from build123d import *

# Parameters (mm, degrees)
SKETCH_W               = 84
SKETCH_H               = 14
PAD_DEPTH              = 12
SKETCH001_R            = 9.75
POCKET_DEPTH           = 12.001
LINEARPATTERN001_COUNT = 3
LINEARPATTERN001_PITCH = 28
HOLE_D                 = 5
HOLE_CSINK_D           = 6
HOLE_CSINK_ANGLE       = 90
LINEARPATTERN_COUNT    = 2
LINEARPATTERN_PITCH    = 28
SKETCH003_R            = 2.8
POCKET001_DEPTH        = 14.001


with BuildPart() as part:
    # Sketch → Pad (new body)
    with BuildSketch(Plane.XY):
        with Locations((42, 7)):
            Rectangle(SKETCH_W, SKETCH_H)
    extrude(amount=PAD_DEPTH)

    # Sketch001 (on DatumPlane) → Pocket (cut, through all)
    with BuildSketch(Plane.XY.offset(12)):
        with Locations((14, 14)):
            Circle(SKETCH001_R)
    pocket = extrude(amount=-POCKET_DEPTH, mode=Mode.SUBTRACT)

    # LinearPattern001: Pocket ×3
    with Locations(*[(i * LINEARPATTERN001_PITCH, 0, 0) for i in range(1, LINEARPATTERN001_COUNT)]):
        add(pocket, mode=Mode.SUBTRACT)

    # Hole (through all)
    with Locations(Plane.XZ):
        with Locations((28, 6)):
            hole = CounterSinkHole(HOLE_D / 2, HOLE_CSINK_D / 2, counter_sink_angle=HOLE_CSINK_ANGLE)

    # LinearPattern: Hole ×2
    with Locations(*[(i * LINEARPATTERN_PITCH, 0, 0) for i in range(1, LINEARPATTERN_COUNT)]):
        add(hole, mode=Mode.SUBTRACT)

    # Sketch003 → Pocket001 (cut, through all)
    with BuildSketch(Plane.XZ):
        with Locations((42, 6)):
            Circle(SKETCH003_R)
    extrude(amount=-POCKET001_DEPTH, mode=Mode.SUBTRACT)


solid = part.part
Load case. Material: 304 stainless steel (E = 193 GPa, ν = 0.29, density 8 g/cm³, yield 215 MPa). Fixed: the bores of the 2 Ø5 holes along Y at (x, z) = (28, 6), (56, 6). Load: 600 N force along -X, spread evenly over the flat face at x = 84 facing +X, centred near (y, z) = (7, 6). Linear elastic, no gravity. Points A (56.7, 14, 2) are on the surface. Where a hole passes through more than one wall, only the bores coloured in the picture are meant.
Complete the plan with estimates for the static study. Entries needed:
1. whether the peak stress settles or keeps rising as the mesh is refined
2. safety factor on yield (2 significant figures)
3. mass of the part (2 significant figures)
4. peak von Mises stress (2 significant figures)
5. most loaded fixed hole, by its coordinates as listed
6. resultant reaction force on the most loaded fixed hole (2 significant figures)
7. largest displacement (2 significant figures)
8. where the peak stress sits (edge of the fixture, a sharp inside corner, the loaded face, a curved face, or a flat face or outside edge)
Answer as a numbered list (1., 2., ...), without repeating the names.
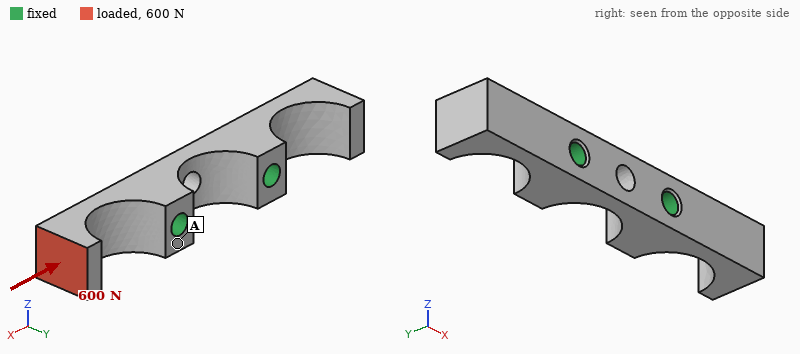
1. settles
2. 2.2
3. 65 g
4. 98 MPa
5. (56, 6)
6. 590 N
7. 38 µm
8. a curved face
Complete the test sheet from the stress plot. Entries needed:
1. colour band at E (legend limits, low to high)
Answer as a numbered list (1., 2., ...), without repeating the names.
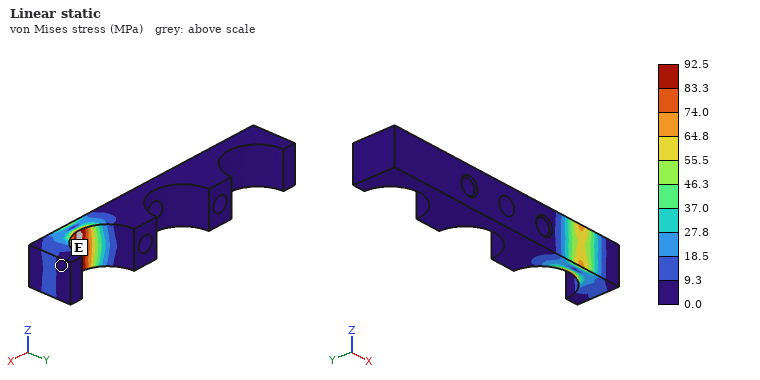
1. 0.0 to 9.3 MPa
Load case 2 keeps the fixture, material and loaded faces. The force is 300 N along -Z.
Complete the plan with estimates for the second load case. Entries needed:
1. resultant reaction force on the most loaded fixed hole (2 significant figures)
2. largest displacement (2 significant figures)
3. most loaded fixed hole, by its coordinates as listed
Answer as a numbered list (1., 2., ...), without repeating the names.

1. 340 N
2. 26 µm
3. (56, 6)
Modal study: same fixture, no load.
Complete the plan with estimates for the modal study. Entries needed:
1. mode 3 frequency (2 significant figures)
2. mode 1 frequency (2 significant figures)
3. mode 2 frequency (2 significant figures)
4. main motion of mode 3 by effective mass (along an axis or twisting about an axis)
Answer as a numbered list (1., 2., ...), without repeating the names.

1. 7200 Hz
2. 4600 Hz
3. 4600 Hz
4. along Z
